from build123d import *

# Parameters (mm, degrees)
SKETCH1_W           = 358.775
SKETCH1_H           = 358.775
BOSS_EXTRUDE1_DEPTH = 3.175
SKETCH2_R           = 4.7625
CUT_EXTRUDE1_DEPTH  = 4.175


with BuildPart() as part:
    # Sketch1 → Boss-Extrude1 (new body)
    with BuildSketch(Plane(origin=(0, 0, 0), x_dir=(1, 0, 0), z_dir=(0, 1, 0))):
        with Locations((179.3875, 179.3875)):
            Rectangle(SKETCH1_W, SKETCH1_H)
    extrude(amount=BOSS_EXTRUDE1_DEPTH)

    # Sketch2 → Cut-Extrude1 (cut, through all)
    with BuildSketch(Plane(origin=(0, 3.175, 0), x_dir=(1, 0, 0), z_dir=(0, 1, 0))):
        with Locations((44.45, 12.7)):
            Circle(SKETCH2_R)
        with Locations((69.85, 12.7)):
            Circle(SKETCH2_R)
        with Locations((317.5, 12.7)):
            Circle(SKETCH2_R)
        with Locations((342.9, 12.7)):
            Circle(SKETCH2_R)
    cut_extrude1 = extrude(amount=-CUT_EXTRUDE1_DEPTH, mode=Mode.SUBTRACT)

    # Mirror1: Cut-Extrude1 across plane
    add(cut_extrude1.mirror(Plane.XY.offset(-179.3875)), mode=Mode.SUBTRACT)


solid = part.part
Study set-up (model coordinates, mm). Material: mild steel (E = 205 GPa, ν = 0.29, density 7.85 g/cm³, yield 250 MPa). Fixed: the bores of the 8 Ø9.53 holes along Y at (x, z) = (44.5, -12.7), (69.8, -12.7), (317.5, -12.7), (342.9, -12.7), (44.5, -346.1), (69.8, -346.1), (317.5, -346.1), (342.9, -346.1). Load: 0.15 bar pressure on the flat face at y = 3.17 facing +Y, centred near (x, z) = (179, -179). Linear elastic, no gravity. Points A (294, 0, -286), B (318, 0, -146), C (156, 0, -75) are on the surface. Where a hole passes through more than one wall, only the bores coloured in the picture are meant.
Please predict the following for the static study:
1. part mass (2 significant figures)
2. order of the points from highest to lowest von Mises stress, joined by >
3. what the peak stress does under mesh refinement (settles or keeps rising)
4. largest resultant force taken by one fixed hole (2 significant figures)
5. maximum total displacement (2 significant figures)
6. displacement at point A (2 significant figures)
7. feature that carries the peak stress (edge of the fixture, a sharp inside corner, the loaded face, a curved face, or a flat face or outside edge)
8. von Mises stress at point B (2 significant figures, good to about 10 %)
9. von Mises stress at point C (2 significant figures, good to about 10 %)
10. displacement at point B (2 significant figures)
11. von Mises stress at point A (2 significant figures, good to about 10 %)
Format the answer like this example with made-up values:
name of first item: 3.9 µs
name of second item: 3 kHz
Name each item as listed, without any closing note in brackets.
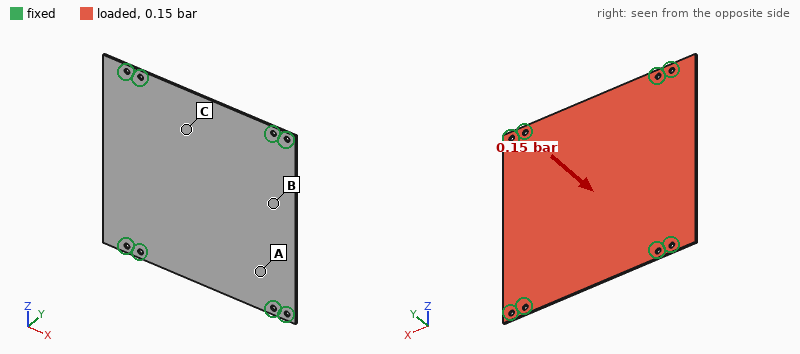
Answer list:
part mass: 3.2 kg
order of the points from highest to lowest von Mises stress, joined by >: B > C > A
what the peak stress does under mesh refinement: keeps rising
largest resultant force taken by one fixed hole: 490 N
maximum total displacement: 1.5 mm
displacement at point A: 0.58 mm
feature that carries the peak stress: edge of the fixture
von Mises stress at point B: 45 MPa
von Mises stress at point C: 25 MPa
displacement at point B: 1.1 mm
von Mises stress at point A: 13 MPa
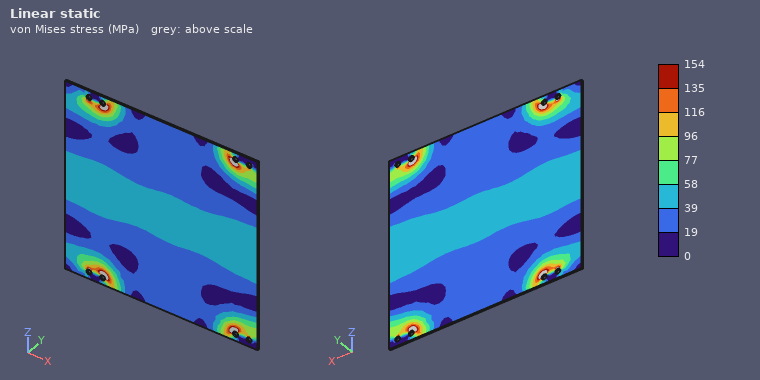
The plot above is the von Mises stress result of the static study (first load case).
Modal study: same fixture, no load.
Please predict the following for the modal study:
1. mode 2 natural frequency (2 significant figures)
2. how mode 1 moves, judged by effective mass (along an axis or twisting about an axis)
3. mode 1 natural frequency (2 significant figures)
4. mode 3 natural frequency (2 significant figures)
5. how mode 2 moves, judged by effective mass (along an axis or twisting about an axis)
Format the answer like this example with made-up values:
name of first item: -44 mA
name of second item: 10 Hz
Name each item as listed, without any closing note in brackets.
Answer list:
mode 2 natural frequency: 170 Hz
how mode 1 moves, judged by effective mass: along Y
mode 1 natural frequency: 120 Hz
mode 3 natural frequency: 230 Hz
how mode 2 moves, judged by effective mass: twisting about Z
